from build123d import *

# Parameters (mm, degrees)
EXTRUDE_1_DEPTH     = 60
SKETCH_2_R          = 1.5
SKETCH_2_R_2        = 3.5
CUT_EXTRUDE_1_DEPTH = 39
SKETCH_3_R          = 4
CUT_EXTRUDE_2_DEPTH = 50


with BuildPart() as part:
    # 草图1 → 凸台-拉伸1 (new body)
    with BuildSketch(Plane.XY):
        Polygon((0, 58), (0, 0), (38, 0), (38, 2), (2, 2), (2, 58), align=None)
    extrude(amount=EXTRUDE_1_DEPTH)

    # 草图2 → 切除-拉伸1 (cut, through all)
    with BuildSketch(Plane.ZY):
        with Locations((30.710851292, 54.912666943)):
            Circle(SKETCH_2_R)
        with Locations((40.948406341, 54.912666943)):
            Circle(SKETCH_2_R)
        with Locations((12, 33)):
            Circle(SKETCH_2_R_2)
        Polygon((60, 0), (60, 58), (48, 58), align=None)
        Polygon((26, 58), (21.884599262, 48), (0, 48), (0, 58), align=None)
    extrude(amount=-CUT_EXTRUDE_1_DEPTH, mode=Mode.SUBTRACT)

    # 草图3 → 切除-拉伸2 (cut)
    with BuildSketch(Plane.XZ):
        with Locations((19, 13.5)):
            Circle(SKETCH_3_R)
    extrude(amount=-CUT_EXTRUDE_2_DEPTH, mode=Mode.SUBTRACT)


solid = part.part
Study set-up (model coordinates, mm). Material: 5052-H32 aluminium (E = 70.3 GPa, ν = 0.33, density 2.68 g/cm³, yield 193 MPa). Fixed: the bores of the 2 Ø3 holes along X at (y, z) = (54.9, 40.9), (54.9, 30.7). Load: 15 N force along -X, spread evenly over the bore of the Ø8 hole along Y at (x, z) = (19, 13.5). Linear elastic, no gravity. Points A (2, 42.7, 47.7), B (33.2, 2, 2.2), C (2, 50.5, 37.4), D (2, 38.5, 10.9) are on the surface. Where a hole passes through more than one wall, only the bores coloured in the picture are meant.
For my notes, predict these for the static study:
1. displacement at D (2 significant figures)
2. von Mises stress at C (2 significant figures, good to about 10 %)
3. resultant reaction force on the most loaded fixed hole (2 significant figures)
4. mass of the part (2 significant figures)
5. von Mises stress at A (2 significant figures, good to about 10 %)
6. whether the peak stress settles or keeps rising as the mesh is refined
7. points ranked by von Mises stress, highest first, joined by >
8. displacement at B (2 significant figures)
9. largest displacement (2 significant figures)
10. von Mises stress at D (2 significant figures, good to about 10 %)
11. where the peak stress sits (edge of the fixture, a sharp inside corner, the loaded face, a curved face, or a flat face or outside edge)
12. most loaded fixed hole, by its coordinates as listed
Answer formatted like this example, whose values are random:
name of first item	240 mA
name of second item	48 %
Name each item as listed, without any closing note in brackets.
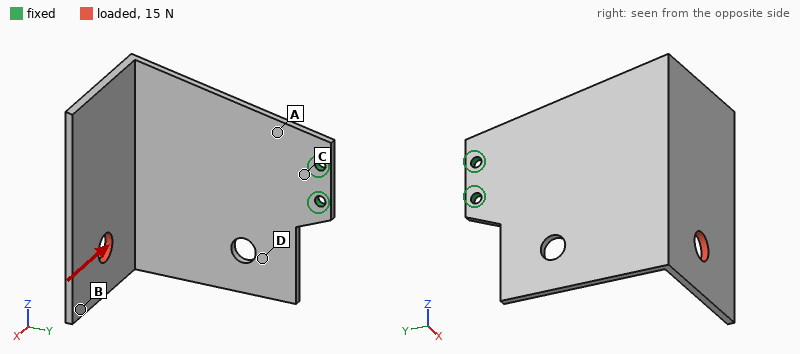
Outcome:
displacement at D	0.13 mm
von Mises stress at C	38 MPa
resultant reaction force on the most loaded fixed hole	29 N
mass of the part	26 g
von Mises stress at A	29 MPa
whether the peak stress settles or keeps rising as the mesh is refined	keeps rising
points ranked by von Mises stress, highest first, joined by >	C > A > D > B
displacement at B	0.77 mm
largest displacement	0.83 mm
von Mises stress at D	11 MPa
where the peak stress sits	edge of the fixture
most loaded fixed hole, by its coordinates as listed	(54.9, 30.7)
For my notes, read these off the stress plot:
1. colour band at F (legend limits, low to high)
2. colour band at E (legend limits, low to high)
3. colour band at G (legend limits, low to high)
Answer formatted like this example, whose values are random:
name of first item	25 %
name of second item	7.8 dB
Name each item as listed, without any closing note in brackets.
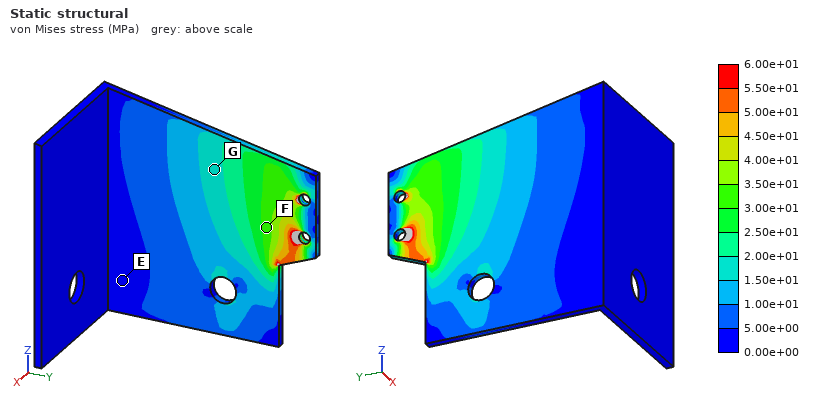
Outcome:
colour band at F	3.00e+01 to 3.50e+01 MPa
colour band at E	0.00e+00 to 5.00e+00 MPa
colour band at G	1.50e+01 to 2.00e+01 MPa
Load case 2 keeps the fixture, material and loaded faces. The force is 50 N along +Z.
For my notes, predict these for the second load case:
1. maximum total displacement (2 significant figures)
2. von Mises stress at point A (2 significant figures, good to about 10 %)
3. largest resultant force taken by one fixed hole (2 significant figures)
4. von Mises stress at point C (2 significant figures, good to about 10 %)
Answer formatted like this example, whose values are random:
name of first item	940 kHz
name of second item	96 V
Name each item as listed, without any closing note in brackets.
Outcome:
maximum total displacement	0.72 mm
von Mises stress at point A	28 MPa
largest resultant force taken by one fixed hole	220 N
von Mises stress at point C	33 MPa
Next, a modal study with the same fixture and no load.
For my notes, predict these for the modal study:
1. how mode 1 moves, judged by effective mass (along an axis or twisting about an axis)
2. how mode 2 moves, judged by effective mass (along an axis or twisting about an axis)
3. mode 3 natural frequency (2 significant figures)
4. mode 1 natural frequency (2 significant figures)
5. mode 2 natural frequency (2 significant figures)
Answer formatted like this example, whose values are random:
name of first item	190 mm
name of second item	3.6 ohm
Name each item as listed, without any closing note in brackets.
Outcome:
how mode 1 moves, judged by effective mass	along X
how mode 2 moves, judged by effective mass	along Z
mode 3 natural frequency	800 Hz
mode 1 natural frequency	200 Hz
mode 2 natural frequency	390 Hz
